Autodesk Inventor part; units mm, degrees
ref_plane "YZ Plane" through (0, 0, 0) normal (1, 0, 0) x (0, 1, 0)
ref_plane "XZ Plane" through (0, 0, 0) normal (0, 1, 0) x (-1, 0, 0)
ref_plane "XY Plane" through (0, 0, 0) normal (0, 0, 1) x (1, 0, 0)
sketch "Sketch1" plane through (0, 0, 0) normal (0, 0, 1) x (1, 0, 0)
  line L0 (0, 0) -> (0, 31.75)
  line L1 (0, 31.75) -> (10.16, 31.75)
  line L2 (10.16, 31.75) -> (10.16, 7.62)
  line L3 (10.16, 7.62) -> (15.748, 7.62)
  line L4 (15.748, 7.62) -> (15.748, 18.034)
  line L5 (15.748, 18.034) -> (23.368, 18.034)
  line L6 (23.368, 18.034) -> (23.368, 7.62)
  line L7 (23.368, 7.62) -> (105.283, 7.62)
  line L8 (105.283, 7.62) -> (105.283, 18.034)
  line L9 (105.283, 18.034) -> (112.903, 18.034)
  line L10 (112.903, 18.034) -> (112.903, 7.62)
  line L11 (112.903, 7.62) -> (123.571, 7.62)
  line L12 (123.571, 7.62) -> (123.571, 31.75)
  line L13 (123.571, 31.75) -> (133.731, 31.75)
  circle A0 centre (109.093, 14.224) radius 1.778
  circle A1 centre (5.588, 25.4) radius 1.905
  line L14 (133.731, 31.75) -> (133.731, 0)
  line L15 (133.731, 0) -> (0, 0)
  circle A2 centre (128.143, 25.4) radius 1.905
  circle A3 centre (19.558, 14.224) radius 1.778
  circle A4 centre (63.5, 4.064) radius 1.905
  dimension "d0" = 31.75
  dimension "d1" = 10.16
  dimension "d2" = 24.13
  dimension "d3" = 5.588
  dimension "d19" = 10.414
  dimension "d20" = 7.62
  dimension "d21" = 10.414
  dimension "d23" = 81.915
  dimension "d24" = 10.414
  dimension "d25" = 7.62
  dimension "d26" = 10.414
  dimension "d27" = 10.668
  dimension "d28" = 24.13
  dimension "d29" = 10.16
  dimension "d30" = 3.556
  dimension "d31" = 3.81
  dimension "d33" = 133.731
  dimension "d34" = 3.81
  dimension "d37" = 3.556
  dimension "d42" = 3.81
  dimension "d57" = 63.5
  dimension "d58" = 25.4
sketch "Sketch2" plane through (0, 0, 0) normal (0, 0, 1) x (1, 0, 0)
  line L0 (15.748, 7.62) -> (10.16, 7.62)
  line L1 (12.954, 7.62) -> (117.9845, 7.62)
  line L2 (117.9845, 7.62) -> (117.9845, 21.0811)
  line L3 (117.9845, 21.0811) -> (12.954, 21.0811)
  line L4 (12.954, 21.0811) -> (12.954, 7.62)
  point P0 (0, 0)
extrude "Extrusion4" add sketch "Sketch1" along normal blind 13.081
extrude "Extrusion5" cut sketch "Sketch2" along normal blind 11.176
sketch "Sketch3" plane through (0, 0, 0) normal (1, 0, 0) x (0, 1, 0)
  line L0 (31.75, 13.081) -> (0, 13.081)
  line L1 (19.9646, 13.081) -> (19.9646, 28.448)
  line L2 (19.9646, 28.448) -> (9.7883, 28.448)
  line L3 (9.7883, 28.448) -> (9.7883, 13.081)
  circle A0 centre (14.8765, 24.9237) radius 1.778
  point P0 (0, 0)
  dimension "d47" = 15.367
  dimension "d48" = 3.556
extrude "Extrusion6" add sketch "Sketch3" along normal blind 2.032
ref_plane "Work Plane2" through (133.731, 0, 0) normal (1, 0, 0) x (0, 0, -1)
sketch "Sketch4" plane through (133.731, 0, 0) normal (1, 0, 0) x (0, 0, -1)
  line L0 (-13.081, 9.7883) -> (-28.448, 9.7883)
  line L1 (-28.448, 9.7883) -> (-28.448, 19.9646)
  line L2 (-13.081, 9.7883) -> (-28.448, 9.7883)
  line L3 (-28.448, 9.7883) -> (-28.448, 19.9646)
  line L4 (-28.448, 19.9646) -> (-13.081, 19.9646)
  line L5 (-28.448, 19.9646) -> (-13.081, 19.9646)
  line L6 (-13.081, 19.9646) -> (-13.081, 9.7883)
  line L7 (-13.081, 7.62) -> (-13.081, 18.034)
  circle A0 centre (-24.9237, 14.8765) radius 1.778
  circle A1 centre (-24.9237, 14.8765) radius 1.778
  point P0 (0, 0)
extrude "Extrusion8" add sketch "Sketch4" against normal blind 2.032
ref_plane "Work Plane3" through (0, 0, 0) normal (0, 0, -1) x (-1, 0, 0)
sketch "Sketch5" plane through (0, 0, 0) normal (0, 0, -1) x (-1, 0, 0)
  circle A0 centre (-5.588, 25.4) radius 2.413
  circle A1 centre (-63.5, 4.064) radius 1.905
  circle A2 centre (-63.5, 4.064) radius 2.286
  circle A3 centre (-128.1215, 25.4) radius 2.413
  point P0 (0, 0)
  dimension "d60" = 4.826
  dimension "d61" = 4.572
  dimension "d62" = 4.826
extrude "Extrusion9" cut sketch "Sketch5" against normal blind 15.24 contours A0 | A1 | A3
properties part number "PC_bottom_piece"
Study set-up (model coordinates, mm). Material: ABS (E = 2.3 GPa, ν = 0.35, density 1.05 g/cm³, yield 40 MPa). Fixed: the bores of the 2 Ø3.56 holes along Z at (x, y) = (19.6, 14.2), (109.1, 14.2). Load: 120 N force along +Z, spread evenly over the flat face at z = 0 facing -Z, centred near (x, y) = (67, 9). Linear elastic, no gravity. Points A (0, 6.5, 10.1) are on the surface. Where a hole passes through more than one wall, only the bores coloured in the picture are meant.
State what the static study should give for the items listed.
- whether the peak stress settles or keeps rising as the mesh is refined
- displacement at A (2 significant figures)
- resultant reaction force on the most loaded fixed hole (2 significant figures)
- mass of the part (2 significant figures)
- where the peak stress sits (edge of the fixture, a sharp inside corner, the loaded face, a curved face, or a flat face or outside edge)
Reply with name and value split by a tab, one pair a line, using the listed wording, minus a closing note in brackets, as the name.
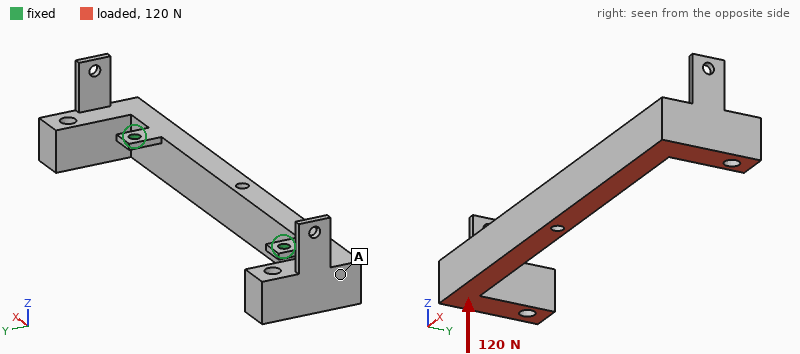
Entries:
whether the peak stress settles or keeps rising as the mesh is refined	keeps rising
displacement at A	0.33 mm
resultant reaction force on the most loaded fixed hole	63 N
mass of the part	21 g
where the peak stress sits	edge of the fixture
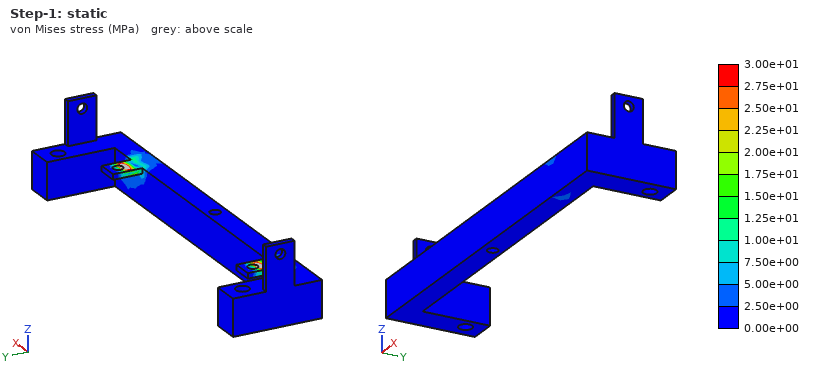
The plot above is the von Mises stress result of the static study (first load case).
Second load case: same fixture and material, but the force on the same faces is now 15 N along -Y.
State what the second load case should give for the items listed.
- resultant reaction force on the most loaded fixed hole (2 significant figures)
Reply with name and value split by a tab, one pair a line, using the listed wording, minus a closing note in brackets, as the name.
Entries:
resultant reaction force on the most loaded fixed hole	7.9 N
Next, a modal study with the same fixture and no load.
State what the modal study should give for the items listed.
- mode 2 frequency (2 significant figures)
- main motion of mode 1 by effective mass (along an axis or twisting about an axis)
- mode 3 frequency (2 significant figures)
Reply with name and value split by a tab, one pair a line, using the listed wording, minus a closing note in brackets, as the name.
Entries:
mode 2 frequency	570 Hz
main motion of mode 1 by effective mass	along Y
mode 3 frequency	670 Hz
